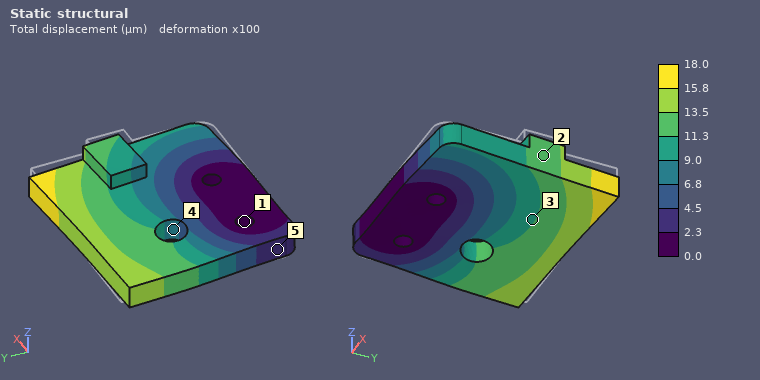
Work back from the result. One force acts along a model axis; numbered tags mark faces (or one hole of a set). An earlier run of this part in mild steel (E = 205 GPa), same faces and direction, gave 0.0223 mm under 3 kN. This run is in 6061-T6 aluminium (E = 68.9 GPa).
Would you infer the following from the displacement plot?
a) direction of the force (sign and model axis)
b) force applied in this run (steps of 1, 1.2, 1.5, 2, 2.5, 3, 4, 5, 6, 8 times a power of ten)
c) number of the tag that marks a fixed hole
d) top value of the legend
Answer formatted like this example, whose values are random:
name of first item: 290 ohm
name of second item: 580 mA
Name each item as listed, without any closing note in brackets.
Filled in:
direction of the force: -X
force applied in this run: 800 N
number of the tag that marks a fixed hole: 1
top value of the legend: 18.0 µm
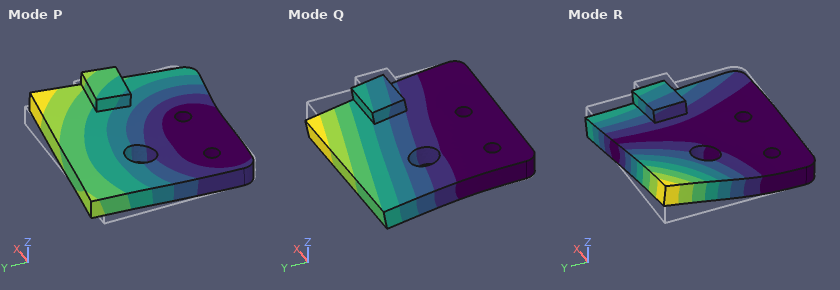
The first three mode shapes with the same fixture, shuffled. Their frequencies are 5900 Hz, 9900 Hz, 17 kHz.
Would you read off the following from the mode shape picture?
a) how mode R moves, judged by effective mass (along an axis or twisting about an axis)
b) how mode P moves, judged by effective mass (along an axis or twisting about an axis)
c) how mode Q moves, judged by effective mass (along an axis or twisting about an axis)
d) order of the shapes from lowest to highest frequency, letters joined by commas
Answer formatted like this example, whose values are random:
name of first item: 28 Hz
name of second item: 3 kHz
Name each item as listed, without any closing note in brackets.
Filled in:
how mode R moves, judged by effective mass: twisting about Y
how mode P moves, judged by effective mass: along X
how mode Q moves, judged by effective mass: along Z
order of the shapes from lowest to highest frequency, letters joined by commas: Q, R, P
